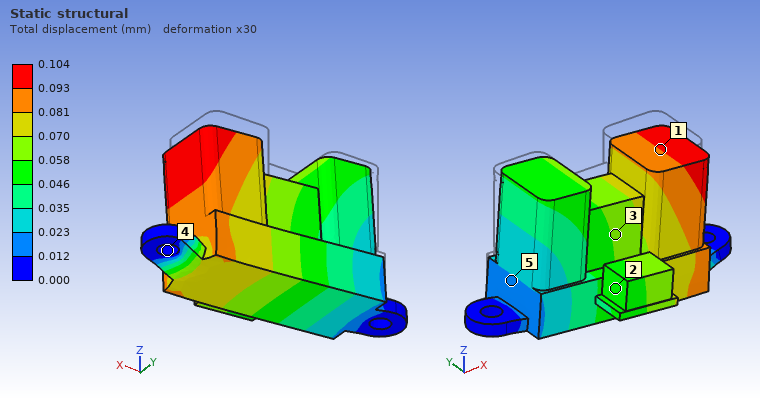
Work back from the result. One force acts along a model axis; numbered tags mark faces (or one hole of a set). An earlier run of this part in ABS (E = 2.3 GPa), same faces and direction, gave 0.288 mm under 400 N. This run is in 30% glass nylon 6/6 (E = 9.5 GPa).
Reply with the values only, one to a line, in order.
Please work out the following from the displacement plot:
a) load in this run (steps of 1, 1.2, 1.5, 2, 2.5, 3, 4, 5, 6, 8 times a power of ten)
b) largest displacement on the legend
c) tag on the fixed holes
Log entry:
600 N
0.104 mm
4
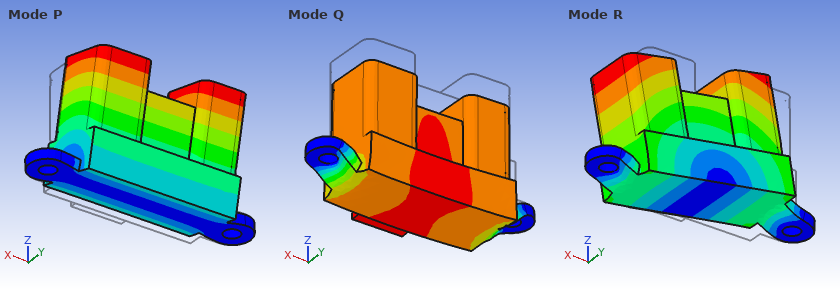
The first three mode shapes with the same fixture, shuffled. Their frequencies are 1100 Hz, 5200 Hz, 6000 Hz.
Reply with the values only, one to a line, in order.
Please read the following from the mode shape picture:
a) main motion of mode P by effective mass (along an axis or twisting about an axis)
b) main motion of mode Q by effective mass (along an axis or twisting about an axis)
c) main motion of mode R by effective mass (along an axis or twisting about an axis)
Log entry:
along Y
along Z
along X
